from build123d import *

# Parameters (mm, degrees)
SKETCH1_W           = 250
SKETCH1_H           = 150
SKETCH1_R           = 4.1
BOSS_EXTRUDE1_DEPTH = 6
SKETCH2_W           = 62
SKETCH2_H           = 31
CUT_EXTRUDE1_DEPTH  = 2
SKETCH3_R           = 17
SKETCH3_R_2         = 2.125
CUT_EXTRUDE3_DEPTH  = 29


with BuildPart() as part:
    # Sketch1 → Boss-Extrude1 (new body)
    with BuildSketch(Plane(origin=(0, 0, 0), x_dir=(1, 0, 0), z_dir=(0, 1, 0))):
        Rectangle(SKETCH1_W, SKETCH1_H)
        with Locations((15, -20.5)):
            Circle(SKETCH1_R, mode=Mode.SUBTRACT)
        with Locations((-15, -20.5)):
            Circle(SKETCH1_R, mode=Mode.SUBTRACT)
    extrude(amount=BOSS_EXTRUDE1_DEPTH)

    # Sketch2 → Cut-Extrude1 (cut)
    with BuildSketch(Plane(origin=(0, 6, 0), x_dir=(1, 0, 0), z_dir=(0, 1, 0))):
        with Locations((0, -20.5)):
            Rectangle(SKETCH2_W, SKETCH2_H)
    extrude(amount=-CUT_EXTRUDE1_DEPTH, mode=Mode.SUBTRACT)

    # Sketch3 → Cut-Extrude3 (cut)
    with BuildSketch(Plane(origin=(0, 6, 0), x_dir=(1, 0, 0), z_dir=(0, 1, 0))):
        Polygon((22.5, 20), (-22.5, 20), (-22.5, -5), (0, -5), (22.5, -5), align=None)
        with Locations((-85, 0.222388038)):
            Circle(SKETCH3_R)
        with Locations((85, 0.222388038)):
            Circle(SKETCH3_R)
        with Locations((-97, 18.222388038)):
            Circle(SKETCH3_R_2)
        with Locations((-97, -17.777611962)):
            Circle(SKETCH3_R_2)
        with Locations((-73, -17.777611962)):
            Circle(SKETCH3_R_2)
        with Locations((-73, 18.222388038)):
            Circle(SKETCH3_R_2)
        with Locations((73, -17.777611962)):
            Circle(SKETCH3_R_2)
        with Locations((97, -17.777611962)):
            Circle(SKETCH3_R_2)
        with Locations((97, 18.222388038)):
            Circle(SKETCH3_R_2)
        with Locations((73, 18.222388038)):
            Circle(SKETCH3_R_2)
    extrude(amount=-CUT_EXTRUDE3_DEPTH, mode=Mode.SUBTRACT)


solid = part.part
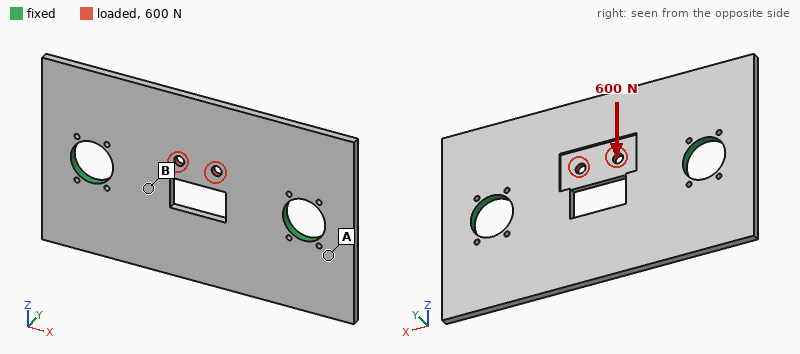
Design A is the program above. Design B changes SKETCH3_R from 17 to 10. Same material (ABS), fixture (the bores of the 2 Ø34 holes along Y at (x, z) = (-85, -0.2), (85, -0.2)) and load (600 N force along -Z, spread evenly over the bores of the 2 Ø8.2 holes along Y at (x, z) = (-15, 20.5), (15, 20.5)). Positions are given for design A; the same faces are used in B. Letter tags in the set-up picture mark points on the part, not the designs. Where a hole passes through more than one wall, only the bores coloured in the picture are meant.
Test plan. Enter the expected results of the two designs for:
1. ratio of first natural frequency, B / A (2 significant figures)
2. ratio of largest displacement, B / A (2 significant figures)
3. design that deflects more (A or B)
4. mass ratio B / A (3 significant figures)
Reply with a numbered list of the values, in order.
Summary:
1. 0.81
2. 1.3
3. B
4. 1.04
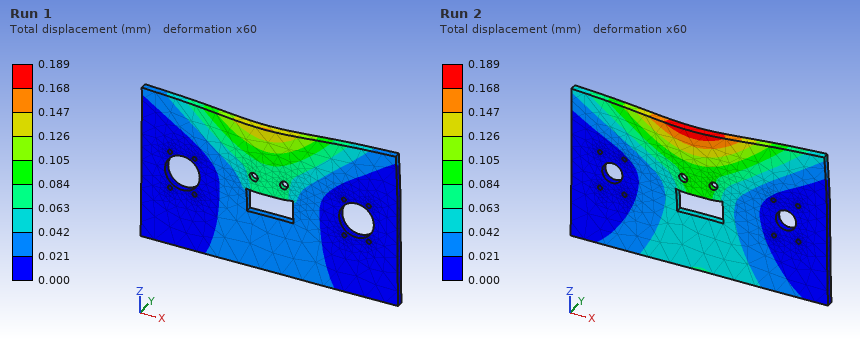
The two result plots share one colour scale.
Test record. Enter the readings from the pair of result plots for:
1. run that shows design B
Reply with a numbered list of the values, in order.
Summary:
1. Run 2
